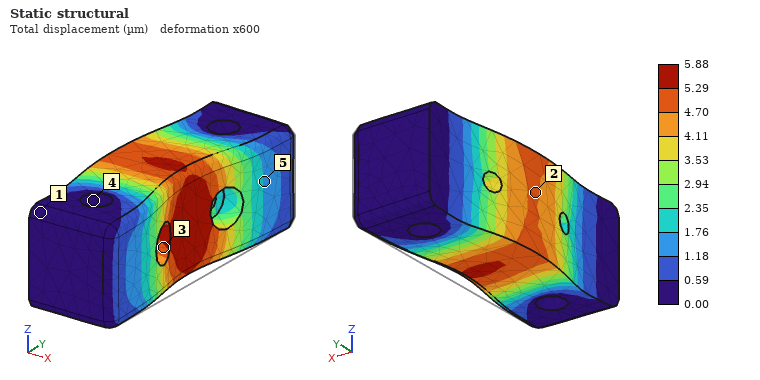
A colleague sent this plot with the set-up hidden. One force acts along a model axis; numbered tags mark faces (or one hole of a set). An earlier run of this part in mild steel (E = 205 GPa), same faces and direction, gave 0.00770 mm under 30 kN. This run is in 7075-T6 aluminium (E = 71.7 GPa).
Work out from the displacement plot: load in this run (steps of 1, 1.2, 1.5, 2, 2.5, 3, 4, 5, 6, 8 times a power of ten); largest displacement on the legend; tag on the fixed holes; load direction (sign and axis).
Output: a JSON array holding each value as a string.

["8 kN", "5.88 µm", "4", "-X"]
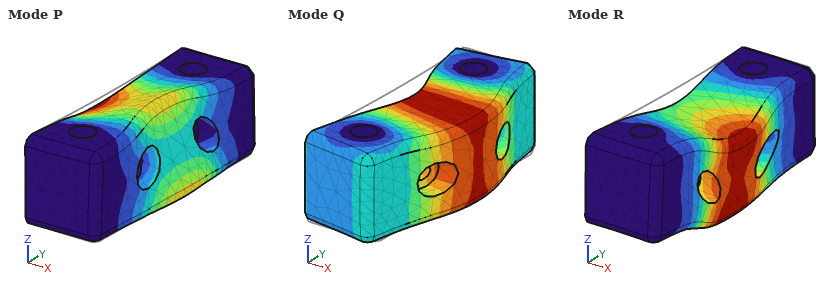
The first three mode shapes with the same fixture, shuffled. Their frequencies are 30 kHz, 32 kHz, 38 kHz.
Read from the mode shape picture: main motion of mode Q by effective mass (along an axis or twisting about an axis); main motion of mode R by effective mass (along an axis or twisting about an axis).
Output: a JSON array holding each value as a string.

["along X", "along Z"]
